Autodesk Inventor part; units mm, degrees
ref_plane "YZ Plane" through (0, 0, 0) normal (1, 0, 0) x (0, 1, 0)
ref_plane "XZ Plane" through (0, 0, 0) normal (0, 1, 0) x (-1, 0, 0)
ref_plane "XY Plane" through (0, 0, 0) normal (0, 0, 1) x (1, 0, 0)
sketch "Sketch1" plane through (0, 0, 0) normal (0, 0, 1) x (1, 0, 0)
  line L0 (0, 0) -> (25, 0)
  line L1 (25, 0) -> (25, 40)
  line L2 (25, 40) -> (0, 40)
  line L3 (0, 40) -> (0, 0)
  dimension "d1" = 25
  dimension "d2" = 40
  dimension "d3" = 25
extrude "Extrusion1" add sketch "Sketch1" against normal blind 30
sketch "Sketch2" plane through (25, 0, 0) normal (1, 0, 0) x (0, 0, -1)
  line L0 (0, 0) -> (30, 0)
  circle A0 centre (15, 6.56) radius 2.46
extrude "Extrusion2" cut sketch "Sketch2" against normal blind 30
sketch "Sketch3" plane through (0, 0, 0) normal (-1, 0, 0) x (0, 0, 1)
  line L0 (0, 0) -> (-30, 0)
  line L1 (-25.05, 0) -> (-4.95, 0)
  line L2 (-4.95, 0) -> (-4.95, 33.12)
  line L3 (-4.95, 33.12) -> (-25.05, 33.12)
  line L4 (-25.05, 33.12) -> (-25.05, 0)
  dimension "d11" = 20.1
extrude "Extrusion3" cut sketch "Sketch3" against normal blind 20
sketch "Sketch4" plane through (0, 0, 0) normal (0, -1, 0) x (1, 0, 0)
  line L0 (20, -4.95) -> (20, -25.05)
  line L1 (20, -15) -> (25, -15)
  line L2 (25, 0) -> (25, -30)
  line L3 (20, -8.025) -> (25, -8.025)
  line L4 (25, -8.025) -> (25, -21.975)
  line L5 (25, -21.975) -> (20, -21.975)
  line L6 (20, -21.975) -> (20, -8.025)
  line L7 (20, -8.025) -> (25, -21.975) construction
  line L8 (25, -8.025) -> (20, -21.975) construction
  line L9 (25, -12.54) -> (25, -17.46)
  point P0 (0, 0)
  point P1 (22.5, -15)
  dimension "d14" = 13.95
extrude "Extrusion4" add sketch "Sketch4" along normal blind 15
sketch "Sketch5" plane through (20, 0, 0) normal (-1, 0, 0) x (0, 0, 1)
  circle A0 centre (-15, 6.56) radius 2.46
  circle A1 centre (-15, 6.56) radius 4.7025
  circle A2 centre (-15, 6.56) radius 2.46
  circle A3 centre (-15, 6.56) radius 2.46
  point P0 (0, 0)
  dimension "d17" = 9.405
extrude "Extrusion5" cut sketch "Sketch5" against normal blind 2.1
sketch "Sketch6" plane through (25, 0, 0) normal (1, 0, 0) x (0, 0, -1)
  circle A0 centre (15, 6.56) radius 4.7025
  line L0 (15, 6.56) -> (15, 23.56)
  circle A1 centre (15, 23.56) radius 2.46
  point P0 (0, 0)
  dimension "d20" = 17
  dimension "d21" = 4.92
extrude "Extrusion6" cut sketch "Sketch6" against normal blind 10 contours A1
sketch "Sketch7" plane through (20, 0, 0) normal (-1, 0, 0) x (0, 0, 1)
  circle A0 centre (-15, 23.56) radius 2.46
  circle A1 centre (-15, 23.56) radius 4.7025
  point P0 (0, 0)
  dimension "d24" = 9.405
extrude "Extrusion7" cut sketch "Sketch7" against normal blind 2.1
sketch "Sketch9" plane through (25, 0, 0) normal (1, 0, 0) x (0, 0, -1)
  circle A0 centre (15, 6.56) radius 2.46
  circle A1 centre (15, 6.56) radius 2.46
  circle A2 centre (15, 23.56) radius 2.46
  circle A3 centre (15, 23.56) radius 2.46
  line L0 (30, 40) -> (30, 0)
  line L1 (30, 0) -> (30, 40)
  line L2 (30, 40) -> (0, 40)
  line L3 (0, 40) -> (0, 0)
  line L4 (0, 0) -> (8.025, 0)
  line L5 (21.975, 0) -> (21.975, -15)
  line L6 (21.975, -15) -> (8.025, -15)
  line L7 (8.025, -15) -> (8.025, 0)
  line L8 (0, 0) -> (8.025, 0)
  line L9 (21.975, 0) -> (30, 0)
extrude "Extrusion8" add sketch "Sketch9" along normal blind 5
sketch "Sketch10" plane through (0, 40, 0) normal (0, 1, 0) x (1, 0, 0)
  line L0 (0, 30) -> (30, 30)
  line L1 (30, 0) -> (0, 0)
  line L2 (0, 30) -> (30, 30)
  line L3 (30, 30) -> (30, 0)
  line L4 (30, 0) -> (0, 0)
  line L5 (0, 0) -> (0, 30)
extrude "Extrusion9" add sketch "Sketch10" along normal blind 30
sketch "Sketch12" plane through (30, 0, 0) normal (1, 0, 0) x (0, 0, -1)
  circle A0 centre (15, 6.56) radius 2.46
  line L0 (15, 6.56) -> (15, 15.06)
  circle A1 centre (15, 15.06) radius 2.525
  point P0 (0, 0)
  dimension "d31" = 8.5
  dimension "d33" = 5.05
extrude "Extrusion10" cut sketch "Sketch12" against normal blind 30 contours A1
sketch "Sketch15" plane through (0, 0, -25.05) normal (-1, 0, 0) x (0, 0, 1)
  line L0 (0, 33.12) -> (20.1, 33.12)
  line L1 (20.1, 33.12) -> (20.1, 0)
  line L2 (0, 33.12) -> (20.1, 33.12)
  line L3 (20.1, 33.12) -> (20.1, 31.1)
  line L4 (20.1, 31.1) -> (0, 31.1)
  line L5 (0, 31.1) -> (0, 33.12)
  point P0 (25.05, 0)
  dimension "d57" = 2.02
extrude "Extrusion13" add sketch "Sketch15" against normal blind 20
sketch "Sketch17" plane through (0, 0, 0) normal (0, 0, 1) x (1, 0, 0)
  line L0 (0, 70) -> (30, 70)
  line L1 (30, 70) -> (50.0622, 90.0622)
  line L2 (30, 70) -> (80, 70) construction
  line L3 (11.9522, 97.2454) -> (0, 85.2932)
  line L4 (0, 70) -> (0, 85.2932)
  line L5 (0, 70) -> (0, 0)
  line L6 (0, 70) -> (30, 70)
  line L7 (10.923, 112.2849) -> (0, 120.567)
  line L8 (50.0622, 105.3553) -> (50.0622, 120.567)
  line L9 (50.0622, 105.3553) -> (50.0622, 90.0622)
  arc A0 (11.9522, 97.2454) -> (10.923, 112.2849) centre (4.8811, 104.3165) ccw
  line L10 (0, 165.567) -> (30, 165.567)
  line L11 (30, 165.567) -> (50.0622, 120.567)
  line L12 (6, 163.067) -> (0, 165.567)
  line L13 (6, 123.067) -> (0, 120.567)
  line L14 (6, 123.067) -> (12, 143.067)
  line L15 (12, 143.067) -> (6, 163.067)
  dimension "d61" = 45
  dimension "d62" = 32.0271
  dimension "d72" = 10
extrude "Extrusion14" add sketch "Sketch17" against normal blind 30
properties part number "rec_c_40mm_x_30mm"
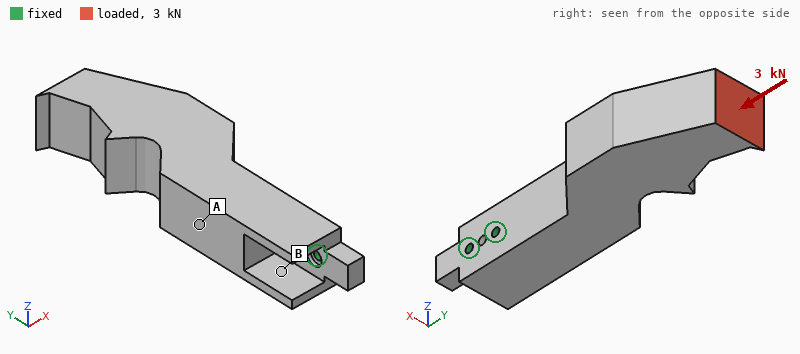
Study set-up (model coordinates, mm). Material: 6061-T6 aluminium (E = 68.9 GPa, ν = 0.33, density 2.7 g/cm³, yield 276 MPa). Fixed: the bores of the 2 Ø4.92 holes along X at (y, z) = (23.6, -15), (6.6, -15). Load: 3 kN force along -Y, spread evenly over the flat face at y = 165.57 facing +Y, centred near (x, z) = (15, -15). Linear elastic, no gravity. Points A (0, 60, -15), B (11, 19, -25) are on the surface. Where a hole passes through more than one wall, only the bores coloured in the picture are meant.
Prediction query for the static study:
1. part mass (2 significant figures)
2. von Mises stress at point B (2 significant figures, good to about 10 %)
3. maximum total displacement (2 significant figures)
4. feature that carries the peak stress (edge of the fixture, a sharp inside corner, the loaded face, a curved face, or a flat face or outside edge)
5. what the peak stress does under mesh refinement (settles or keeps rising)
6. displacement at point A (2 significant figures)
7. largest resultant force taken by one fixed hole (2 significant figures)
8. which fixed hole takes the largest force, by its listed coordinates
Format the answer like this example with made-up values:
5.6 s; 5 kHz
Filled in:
420 g; 11 MPa; 0.14 mm; edge of the fixture; keeps rising; 0.032 mm; 2.3 kN; (23.6, -15)
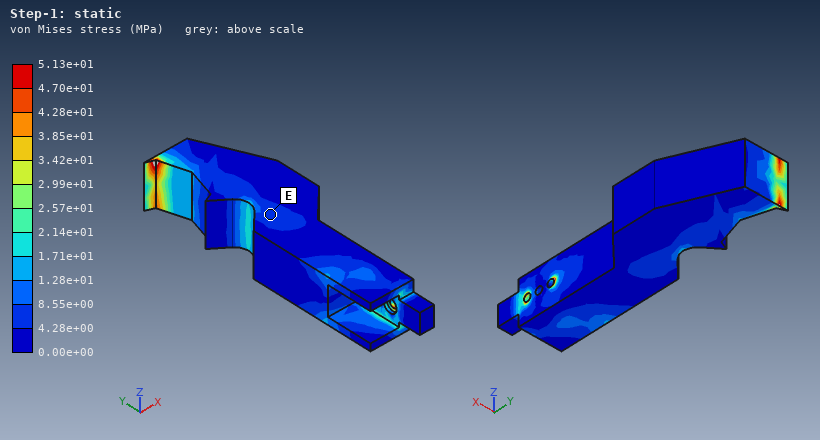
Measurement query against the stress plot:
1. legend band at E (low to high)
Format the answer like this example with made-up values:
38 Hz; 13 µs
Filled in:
4.28e+00 to 8.55e+00 MPa
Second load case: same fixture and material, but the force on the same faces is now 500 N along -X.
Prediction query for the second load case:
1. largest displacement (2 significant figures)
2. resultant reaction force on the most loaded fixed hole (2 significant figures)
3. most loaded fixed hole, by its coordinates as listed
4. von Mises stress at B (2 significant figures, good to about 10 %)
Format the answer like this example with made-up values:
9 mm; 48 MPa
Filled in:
0.32 mm; 3.4 kN; (23.6, -15); 23 MPa
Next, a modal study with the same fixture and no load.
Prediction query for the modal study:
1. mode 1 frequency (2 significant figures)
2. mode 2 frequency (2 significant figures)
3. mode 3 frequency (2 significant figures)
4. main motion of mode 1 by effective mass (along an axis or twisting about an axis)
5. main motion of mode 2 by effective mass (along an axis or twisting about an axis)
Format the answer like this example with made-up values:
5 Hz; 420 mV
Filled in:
580 Hz; 670 Hz; 2200 Hz; along X; along Z
